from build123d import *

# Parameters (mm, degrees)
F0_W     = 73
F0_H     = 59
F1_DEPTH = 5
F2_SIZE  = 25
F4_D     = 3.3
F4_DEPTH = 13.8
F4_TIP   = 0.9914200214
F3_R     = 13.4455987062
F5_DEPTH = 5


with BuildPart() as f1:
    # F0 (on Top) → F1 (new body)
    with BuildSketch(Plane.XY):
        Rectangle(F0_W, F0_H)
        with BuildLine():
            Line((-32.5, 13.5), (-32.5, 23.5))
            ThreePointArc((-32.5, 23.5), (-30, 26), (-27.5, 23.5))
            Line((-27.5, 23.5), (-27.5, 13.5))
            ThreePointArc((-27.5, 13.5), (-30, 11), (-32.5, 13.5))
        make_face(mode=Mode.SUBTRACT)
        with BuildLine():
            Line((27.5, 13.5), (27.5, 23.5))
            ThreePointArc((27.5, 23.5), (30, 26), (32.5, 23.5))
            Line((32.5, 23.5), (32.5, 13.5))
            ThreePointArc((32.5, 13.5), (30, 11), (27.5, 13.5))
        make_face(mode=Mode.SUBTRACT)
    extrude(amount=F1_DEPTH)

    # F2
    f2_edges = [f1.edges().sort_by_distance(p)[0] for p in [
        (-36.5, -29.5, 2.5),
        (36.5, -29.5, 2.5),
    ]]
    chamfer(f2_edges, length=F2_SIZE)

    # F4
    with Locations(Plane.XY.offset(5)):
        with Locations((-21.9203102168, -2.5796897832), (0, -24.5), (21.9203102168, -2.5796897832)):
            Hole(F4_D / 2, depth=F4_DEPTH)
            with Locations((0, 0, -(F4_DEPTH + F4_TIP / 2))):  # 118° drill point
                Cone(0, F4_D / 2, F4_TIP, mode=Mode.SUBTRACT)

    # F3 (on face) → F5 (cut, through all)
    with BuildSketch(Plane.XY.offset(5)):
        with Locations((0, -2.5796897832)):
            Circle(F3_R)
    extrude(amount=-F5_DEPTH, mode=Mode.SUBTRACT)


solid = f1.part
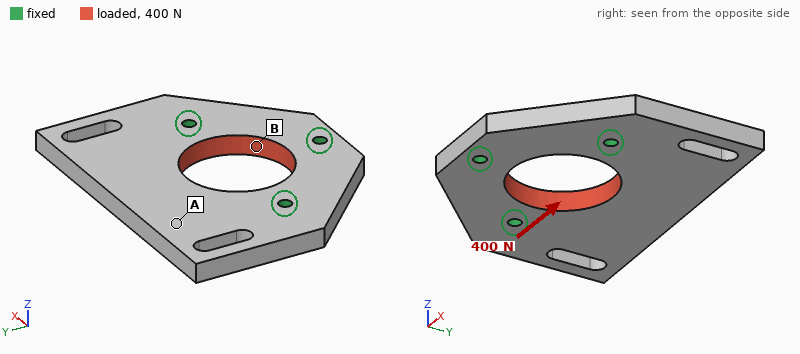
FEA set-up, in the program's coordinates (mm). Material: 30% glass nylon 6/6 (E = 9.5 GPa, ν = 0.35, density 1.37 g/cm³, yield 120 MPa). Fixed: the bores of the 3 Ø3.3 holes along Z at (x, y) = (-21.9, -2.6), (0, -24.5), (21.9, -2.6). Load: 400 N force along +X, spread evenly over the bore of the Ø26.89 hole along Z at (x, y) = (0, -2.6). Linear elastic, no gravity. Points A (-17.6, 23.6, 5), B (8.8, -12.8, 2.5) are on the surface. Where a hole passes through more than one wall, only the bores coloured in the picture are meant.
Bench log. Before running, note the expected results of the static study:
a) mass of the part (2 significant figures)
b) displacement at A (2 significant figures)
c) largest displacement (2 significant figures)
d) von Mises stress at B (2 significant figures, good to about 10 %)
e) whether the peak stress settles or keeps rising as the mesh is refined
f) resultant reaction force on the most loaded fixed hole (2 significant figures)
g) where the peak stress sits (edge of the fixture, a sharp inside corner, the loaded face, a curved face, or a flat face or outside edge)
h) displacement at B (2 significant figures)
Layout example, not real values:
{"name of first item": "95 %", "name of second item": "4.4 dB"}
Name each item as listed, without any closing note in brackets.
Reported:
{"mass of the part": "20 g", "displacement at A": "5.7 µm", "largest displacement": "6.9 µm", "von Mises stress at B": "1.5 MPa", "whether the peak stress settles or keeps rising as the mesh is refined": "keeps rising", "resultant reaction force on the most loaded fixed hole": "160 N", "where the peak stress sits": "edge of the fixture", "displacement at B": "2.6 µm"}
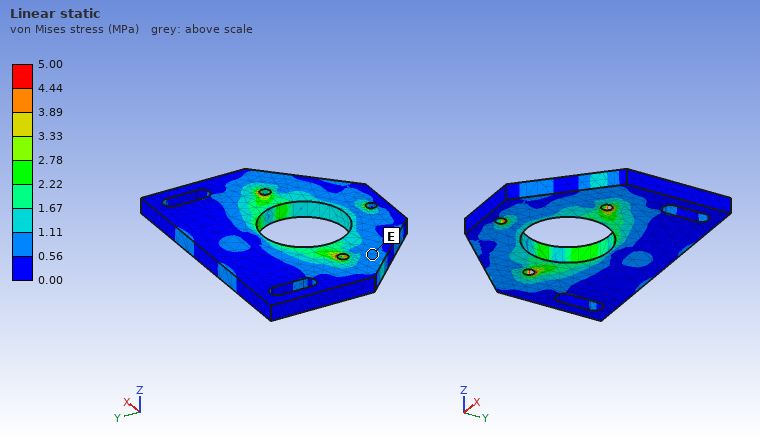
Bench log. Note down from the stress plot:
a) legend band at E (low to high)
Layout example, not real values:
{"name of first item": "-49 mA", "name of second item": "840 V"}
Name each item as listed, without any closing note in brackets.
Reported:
{"legend band at E": "0.56 to 1.11 MPa"}
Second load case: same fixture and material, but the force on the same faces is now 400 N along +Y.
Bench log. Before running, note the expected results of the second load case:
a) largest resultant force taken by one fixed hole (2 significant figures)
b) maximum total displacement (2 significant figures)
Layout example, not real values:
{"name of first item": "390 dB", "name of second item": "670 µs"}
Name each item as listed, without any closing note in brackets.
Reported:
{"largest resultant force taken by one fixed hole": "150 N", "maximum total displacement": "5.7 µm"}
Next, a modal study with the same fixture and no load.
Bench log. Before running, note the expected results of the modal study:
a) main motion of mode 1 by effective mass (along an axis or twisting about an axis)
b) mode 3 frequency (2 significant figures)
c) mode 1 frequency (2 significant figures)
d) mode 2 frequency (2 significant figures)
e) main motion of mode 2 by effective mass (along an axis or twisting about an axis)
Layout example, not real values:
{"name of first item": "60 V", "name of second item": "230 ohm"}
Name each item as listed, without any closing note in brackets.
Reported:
{"main motion of mode 1 by effective mass": "along Z", "mode 3 frequency": "4000 Hz", "mode 1 frequency": "1600 Hz", "mode 2 frequency": "2600 Hz", "main motion of mode 2 by effective mass": "twisting about Y"}
